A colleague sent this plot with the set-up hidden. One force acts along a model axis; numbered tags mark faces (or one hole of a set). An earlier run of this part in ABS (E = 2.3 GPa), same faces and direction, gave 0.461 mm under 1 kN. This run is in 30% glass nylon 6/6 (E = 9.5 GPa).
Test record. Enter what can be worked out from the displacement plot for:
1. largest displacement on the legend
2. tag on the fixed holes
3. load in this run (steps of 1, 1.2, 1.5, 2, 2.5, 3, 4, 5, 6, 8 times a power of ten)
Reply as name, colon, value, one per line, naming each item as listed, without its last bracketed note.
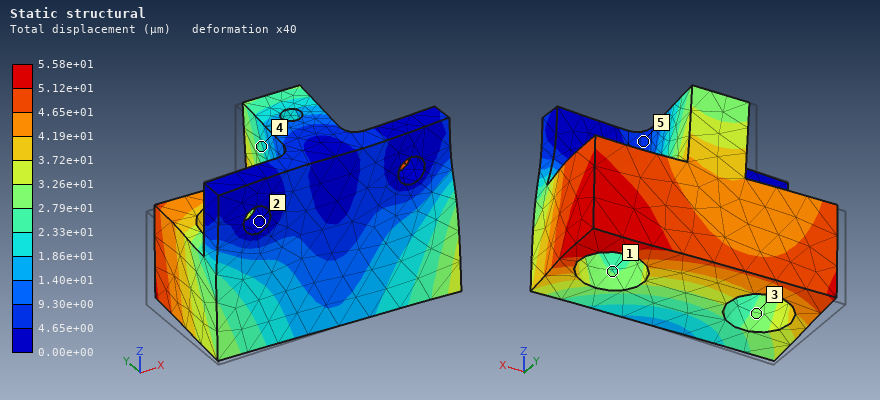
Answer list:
largest displacement on the legend: 5.58e+01 µm
tag on the fixed holes: 2
load in this run: 500 N
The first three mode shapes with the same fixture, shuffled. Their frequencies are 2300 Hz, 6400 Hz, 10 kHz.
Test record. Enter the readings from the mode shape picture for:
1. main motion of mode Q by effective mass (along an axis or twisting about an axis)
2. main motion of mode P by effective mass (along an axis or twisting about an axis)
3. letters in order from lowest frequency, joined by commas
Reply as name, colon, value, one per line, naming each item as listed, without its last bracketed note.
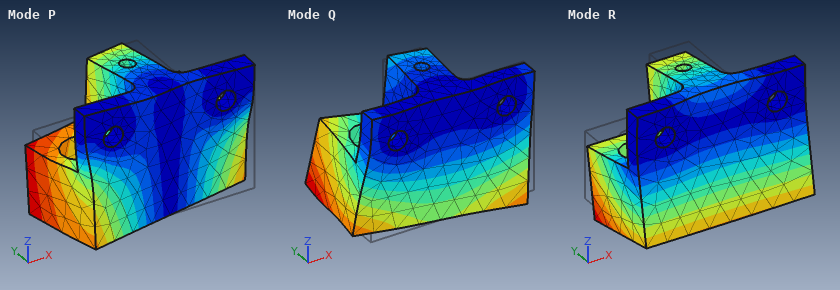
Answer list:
main motion of mode Q by effective mass: along X
main motion of mode P by effective mass: along X
letters in order from lowest frequency, joined by commas: R, P, Q
